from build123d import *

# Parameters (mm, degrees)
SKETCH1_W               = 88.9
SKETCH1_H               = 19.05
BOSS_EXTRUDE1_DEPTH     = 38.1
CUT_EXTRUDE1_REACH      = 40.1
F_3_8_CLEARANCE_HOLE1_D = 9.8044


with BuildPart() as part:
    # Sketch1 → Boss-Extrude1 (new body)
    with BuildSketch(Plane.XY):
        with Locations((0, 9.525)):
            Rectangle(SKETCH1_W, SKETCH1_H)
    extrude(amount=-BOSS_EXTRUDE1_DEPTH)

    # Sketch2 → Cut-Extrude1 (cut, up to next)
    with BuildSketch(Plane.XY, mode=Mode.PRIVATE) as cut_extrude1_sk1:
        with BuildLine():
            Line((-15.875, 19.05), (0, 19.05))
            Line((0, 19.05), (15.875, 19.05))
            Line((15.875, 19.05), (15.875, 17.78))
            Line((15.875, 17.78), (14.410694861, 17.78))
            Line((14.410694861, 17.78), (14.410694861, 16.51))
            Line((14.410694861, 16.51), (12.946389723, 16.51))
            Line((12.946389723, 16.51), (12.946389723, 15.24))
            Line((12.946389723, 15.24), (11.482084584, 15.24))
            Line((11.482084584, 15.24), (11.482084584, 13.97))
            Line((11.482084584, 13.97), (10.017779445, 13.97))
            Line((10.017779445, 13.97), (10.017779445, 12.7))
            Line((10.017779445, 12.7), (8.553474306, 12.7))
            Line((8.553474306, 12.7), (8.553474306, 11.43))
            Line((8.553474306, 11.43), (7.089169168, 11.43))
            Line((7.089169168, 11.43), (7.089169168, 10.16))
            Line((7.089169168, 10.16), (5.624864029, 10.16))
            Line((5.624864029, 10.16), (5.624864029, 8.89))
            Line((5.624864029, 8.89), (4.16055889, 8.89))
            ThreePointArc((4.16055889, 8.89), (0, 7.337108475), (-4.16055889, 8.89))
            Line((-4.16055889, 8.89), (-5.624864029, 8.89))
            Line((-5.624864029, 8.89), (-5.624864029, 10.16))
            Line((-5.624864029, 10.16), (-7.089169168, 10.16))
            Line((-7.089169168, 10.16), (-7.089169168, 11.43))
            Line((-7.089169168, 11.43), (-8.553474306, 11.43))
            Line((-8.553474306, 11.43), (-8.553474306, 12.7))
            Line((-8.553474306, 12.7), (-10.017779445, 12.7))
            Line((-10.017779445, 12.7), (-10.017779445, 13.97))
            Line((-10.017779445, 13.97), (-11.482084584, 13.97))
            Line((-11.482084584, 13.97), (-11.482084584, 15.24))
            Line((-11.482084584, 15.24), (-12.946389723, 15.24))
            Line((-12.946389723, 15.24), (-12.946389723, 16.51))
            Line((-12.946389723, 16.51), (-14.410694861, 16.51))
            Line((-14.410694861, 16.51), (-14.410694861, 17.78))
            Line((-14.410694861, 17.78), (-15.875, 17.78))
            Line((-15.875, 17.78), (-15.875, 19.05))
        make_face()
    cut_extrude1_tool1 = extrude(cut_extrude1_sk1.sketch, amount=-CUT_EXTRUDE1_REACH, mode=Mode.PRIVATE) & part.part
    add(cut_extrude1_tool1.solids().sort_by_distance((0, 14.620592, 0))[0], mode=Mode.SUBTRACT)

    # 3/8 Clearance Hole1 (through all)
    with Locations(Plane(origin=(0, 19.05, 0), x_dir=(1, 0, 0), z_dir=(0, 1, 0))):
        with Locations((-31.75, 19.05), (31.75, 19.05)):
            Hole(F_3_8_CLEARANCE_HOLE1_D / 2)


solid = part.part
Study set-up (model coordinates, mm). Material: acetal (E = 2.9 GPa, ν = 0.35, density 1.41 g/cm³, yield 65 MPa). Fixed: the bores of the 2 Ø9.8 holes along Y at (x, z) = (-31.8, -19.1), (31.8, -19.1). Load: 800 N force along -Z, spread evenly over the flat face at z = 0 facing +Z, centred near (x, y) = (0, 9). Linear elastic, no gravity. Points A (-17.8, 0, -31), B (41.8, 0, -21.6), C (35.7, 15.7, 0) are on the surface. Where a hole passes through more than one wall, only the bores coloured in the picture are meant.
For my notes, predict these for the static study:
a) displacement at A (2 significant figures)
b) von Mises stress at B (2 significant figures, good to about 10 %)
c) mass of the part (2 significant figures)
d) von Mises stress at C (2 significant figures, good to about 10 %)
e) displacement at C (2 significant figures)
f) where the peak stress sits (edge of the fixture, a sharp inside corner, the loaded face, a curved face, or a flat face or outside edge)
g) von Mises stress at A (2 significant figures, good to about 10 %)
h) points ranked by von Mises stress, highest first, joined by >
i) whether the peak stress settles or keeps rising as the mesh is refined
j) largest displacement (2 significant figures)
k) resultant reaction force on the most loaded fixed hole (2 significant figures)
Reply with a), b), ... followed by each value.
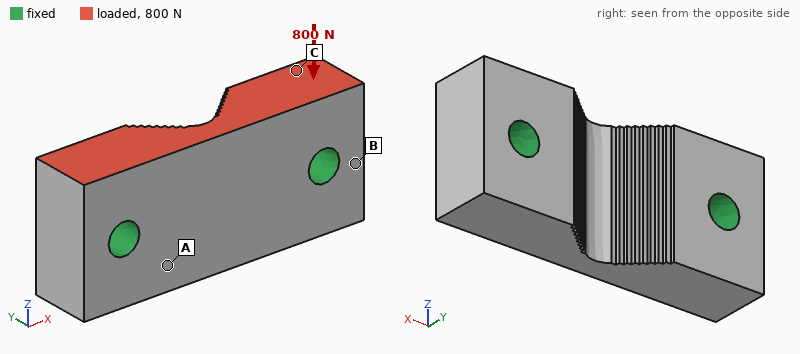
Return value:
a) 6.1 µm
b) 0.25 MPa
c) 75 g
d) 0.70 MPa
e) 3.9 µm
f) edge of the fixture
g) 0.56 MPa
h) C > A > B
i) keeps rising
j) 15 µm
k) 400 N
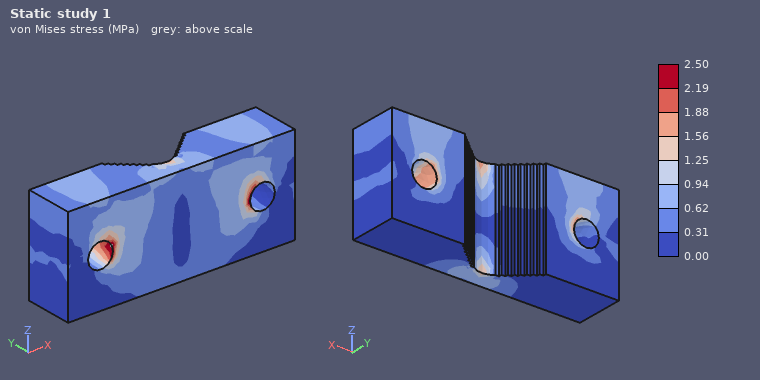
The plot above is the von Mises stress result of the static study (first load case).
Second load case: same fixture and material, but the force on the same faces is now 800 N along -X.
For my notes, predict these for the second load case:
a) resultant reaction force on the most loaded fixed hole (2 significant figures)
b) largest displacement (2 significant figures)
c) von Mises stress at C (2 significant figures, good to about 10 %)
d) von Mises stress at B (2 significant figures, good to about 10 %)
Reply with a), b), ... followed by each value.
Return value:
a) 430 N
b) 22 µm
c) 1.2 MPa
d) 0.65 MPa
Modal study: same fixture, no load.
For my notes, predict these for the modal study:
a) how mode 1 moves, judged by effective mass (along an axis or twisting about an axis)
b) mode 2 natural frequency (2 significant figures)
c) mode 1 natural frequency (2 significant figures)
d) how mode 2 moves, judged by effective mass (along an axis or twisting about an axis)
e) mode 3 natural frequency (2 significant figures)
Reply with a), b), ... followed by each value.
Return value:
a) along Z
b) 5000 Hz
c) 4800 Hz
d) along Y
e) 6200 Hz
